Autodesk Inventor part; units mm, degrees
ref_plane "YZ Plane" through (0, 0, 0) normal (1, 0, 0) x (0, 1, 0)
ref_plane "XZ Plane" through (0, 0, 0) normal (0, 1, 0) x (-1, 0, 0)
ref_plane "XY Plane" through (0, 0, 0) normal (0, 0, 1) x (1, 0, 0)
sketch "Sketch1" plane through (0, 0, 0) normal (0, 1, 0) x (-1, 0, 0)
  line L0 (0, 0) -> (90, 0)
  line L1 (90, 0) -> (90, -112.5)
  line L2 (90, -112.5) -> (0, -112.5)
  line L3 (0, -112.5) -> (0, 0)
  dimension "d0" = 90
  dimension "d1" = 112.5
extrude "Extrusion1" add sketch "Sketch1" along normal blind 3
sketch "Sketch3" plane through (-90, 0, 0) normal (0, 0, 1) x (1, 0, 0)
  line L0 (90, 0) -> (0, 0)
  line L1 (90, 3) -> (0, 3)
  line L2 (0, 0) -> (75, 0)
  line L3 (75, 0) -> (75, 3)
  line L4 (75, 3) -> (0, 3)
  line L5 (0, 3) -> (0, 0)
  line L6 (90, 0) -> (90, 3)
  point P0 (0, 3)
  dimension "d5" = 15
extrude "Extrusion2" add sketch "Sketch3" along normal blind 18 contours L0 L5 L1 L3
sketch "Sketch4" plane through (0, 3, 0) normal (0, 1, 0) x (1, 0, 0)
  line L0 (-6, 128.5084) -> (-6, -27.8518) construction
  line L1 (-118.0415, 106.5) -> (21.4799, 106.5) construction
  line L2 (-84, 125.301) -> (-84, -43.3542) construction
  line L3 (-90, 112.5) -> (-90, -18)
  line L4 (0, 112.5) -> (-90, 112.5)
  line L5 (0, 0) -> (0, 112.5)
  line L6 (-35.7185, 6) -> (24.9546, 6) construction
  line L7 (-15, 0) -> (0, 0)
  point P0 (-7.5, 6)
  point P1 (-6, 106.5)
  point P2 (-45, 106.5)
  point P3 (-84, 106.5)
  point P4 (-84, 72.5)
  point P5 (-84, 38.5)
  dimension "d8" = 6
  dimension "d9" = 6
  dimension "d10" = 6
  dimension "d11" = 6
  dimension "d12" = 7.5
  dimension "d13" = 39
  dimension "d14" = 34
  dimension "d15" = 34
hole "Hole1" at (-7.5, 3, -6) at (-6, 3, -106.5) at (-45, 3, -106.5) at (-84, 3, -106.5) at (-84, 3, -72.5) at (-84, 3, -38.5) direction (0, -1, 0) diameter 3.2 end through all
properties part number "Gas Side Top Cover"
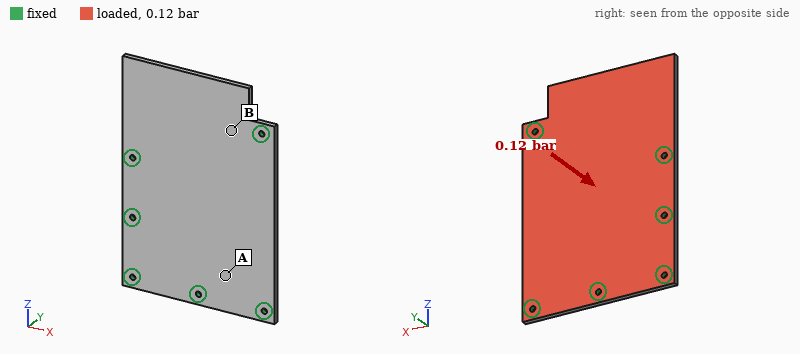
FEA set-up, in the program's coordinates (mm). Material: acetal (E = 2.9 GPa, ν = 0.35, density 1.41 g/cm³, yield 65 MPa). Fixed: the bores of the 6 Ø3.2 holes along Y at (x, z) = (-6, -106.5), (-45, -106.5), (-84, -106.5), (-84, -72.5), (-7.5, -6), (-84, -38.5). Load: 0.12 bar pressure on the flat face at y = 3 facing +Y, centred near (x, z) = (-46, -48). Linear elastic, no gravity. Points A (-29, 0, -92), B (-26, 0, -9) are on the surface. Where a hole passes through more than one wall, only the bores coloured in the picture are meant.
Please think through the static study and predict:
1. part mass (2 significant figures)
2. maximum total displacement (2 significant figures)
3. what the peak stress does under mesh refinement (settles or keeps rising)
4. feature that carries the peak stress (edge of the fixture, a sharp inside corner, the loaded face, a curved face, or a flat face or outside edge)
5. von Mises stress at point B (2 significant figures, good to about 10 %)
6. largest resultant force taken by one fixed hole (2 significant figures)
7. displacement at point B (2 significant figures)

48 g
1.7 mm
keeps rising
edge of the fixture
5.0 MPa
43 N
0.32 mm
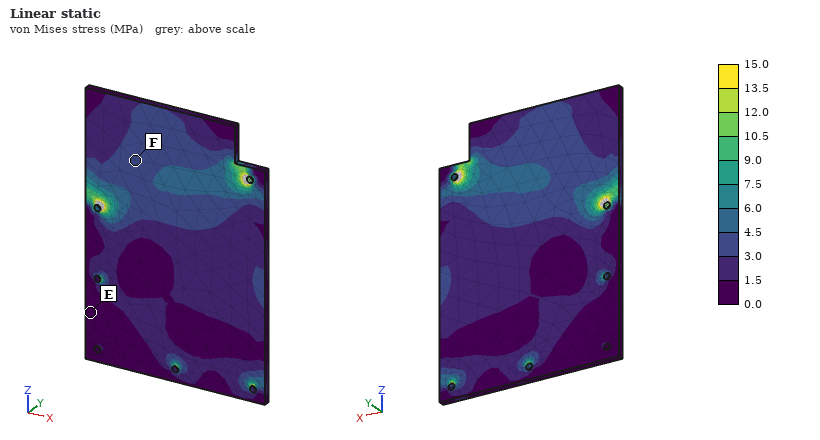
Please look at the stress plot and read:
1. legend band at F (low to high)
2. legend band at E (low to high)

3.0 to 4.5 MPa
0.0 to 1.5 MPa
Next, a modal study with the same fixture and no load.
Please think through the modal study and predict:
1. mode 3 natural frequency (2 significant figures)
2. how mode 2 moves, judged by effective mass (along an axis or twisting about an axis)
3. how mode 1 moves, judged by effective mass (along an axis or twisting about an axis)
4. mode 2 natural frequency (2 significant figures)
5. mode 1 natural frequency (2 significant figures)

670 Hz
along Y
along Y
440 Hz
260 Hz
